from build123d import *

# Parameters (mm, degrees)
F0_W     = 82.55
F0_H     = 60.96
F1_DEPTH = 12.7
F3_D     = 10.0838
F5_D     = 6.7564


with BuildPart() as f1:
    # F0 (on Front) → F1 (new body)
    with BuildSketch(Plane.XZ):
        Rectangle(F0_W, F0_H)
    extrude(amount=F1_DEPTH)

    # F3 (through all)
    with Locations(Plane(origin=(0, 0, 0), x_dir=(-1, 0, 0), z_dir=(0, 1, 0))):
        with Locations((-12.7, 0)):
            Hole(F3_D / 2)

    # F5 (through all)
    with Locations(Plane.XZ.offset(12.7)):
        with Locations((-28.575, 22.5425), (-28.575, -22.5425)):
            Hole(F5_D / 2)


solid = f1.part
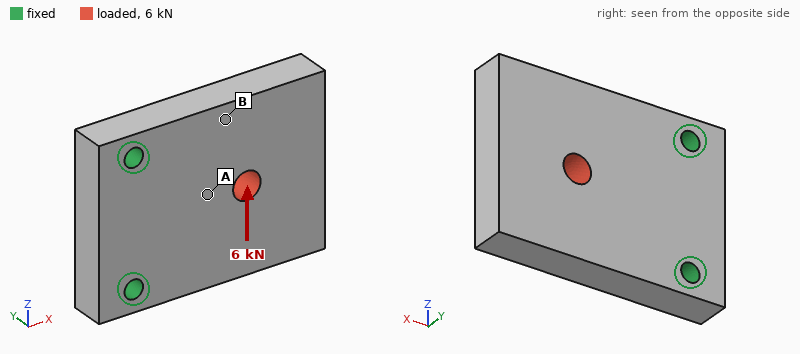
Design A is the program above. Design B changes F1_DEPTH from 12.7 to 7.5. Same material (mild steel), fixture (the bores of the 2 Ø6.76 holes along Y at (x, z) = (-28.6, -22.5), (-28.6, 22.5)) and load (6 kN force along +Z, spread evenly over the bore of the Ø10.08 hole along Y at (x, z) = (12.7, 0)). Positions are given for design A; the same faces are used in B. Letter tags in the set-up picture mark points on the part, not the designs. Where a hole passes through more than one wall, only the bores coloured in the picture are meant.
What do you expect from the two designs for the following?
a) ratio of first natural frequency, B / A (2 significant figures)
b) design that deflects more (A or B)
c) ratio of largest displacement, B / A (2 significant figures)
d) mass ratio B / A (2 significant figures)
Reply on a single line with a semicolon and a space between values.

0.62; B; 1.7; 0.59
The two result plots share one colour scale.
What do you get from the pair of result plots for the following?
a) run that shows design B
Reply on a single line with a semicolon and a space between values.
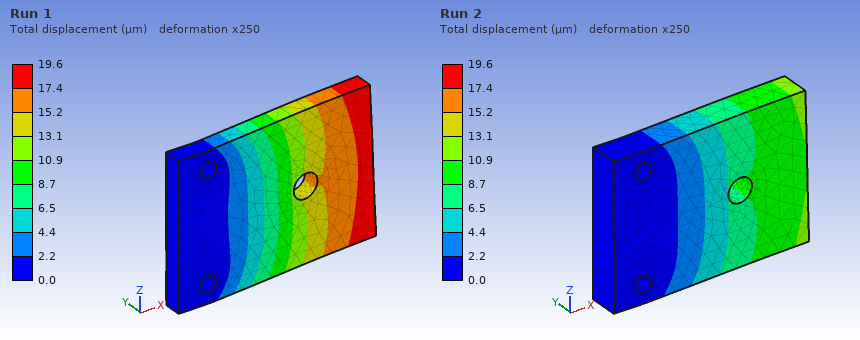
Run 1
